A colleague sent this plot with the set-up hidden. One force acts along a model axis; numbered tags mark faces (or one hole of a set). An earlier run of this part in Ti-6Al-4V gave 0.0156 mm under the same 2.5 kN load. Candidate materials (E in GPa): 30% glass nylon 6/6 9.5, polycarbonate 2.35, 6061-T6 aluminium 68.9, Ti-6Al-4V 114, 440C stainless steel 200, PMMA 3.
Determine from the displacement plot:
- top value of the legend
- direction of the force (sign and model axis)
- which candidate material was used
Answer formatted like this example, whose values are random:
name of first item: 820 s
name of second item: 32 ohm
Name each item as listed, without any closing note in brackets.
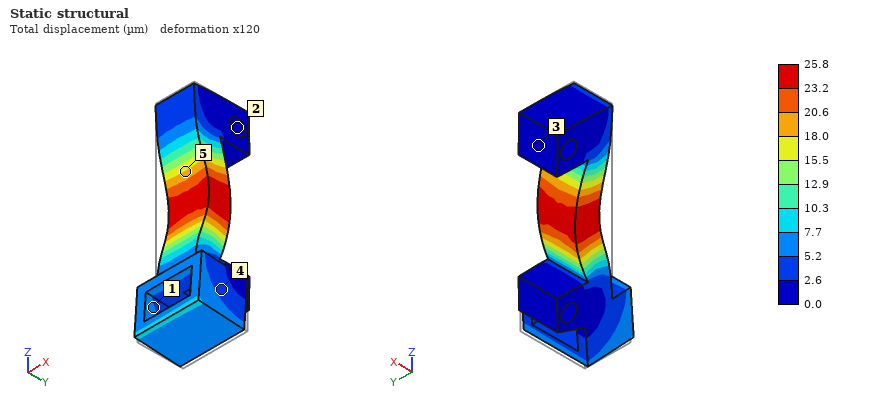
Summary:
top value of the legend: 25.8 µm
direction of the force: +Y
which candidate material was used: 6061-T6 aluminium
